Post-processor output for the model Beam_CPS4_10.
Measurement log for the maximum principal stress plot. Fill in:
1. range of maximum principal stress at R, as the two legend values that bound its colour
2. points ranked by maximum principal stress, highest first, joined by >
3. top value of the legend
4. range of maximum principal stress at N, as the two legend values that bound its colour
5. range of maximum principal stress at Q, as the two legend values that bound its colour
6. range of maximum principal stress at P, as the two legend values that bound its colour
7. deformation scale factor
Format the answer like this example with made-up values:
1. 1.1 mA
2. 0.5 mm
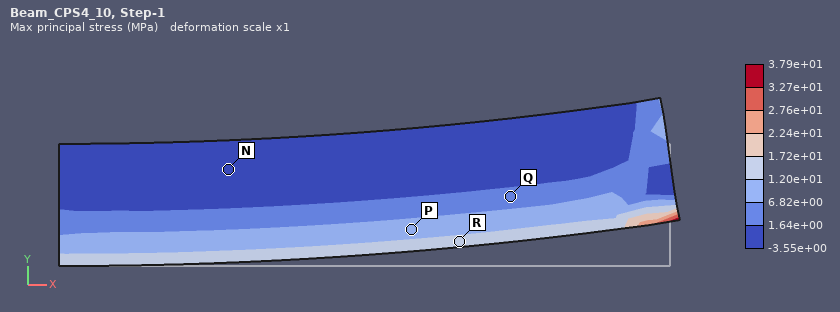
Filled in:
1. 1.20e+01 to 1.72e+01 MPa
2. R > P > Q > N
3. 3.79e+01 MPa
4. -3.55e+00 to 1.64e+00 MPa
5. 1.64e+00 to 6.82e+00 MPa
6. 6.82e+00 to 1.20e+01 MPa
7. 1
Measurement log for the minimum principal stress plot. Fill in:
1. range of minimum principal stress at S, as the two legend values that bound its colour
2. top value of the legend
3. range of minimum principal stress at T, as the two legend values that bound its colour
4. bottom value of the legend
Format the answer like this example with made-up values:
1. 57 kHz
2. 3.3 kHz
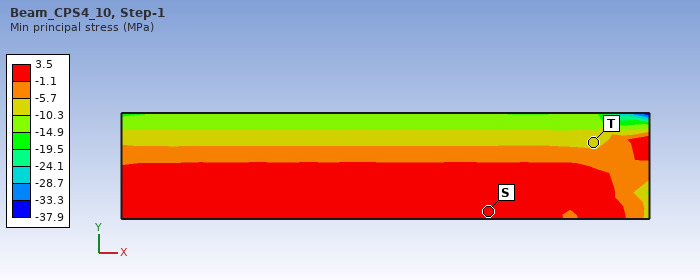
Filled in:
1. -1.1 to 3.5 MPa
2. 3.5 MPa
3. -10.3 to -5.7 MPa
4. -37.9 MPa
